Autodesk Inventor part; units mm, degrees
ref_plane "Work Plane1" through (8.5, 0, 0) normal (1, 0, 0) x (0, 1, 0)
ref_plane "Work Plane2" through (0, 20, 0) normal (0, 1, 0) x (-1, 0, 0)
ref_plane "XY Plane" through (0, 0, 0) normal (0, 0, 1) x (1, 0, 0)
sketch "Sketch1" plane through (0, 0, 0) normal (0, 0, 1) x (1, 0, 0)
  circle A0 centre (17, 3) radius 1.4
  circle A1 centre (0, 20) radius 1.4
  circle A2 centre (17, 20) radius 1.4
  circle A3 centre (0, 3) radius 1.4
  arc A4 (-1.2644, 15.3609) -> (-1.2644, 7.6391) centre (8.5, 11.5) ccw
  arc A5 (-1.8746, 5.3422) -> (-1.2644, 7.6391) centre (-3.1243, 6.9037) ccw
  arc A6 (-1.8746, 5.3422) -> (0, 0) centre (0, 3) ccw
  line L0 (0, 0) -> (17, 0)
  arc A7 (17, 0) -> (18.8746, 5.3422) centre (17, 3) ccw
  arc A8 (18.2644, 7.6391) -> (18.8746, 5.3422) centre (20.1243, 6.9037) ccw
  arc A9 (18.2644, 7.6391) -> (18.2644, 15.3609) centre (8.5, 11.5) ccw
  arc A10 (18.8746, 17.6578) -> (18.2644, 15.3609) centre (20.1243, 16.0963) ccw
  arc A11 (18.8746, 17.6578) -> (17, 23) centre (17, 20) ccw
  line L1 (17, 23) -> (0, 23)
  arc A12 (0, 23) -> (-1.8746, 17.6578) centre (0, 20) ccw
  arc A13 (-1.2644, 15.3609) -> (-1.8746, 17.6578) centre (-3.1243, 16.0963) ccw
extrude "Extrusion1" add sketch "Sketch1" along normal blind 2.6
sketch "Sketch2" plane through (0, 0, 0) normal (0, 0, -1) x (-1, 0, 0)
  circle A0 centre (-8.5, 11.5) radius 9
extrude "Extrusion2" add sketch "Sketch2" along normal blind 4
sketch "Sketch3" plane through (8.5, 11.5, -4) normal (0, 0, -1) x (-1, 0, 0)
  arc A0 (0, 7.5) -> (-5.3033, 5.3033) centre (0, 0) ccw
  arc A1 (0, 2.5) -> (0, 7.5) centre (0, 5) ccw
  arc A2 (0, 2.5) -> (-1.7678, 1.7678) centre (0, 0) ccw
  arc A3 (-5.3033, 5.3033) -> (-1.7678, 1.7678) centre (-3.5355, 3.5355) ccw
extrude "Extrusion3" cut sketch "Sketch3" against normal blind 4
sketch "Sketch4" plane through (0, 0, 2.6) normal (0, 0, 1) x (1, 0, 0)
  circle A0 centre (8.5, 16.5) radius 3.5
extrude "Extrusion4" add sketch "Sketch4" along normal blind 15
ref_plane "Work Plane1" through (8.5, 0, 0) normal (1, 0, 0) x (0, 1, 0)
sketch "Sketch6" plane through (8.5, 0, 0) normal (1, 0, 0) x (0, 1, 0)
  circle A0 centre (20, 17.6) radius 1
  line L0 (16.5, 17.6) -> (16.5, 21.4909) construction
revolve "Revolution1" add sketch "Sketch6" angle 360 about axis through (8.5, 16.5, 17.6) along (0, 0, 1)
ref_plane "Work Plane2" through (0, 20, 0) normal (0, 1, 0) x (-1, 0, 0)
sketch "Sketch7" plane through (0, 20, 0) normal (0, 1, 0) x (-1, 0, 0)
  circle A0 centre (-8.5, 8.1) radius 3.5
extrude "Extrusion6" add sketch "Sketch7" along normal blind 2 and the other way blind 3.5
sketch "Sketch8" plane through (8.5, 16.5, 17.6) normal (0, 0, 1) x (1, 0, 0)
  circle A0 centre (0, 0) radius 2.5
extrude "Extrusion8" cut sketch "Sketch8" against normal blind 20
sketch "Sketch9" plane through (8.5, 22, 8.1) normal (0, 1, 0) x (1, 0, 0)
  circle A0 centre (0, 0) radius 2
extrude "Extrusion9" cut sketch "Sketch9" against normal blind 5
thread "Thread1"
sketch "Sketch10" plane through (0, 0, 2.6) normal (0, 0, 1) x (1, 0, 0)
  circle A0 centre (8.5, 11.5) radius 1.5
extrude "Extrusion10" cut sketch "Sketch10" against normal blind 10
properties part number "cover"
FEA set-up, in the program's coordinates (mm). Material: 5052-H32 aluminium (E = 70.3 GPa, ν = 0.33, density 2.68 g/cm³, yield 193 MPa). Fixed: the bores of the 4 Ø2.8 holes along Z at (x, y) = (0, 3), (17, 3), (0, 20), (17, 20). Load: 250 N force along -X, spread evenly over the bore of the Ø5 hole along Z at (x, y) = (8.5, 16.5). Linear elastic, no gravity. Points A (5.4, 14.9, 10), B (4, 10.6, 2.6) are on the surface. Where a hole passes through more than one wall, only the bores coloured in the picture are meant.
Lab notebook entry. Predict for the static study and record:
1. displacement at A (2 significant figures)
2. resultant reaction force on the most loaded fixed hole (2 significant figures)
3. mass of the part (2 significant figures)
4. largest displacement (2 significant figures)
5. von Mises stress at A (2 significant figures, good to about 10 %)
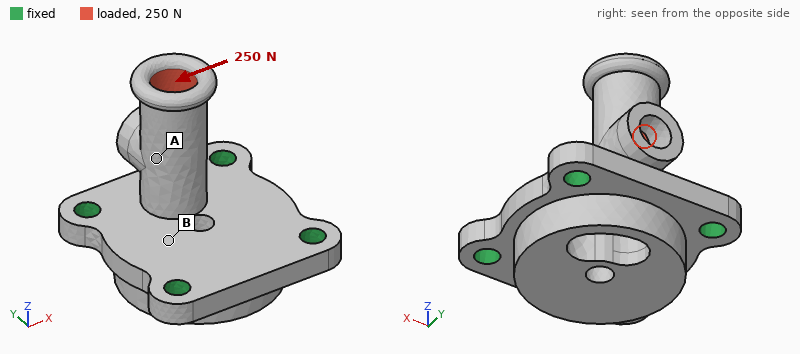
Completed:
18 µm
150 N
6.3 g
37 µm
16 MPa
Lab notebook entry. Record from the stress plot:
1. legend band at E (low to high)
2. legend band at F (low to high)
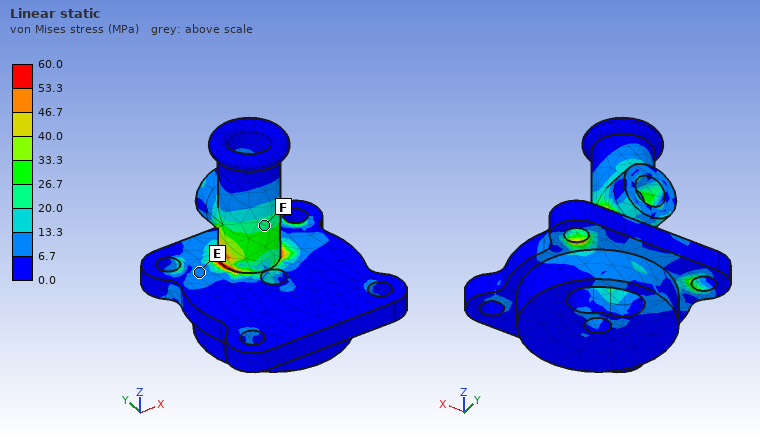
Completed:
6.7 to 13.3 MPa
20.0 to 26.7 MPa
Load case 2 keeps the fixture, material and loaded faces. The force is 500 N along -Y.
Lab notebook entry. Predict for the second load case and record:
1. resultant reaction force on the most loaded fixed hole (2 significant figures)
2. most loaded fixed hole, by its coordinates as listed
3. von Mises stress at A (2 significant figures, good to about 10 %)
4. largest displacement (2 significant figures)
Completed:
240 N
(0, 20)
35 MPa
85 µm
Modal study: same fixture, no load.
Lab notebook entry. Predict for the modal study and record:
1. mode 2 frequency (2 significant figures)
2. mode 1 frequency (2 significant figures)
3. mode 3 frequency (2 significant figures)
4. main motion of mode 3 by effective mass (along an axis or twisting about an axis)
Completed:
13 kHz
12 kHz
31 kHz
along Z
